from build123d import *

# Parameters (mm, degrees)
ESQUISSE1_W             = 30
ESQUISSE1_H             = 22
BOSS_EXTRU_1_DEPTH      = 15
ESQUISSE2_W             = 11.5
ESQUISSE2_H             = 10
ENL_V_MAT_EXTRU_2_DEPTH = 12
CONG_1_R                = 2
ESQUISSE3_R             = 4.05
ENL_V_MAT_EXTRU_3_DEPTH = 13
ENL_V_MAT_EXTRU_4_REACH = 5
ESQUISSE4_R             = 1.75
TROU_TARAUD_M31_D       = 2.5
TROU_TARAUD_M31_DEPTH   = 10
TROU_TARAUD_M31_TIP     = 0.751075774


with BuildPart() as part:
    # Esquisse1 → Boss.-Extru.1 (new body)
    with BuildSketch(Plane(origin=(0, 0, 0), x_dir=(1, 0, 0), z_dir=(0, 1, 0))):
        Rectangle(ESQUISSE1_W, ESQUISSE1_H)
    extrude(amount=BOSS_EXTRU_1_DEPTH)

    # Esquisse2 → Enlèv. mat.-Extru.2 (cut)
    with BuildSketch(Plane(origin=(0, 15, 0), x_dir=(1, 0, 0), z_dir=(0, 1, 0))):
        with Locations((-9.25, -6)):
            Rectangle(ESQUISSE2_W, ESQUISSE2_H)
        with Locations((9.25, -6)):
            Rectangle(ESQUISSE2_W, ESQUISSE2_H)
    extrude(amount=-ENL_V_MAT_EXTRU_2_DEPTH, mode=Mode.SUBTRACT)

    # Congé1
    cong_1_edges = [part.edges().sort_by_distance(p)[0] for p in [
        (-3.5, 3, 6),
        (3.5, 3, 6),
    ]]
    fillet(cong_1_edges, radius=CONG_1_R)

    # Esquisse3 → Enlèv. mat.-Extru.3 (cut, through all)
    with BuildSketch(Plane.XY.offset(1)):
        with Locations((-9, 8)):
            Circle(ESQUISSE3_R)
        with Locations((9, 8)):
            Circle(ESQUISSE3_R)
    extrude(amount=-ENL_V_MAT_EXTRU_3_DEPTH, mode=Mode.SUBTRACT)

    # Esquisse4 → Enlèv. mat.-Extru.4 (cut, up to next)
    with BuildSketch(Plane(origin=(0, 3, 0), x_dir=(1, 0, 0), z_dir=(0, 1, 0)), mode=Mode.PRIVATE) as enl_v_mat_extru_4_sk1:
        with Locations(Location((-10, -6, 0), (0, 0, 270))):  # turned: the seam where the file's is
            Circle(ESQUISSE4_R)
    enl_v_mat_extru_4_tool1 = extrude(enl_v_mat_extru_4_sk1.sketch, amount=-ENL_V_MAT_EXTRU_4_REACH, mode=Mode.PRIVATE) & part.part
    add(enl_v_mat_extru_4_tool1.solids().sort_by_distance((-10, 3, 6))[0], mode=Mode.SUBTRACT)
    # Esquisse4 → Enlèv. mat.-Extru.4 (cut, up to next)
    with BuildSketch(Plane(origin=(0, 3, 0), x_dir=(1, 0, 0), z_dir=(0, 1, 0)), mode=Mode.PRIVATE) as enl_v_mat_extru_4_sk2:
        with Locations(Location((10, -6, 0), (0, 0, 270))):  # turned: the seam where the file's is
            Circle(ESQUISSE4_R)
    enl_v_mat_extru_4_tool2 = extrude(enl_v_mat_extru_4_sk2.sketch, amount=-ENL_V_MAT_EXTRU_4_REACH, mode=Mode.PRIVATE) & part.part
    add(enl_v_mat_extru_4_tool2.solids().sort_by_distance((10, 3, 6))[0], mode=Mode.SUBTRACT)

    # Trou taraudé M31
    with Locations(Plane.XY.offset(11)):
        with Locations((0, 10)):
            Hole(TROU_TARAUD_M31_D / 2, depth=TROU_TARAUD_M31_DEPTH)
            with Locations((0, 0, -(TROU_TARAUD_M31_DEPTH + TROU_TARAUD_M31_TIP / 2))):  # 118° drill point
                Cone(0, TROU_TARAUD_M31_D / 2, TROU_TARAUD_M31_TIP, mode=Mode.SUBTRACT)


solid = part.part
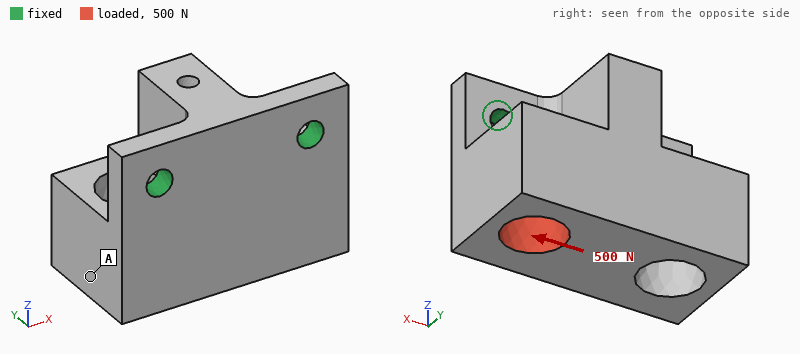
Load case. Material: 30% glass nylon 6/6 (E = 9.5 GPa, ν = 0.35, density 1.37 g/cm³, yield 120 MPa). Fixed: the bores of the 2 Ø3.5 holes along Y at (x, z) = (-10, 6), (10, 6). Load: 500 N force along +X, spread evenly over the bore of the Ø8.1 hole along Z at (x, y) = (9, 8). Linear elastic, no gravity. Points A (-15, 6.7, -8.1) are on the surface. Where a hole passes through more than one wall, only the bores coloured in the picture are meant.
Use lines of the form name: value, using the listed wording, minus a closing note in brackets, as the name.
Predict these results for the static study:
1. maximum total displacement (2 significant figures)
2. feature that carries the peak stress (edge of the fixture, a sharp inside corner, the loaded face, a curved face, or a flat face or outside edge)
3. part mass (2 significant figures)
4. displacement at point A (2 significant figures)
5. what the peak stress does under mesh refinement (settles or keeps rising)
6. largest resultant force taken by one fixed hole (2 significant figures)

maximum total displacement: 56 µm
feature that carries the peak stress: edge of the fixture
part mass: 8.0 g
displacement at point A: 38 µm
what the peak stress does under mesh refinement: keeps rising
largest resultant force taken by one fixed hole: 390 N
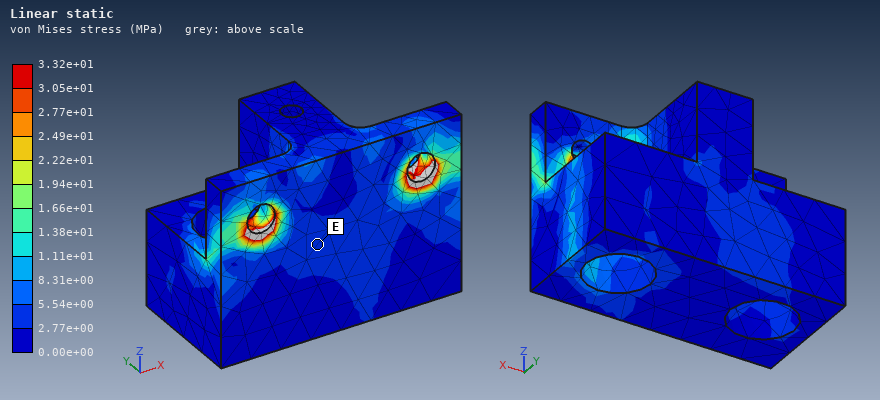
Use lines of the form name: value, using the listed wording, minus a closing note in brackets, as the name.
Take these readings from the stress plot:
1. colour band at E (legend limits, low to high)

colour band at E: 2.77e+00 to 5.54e+00 MPa
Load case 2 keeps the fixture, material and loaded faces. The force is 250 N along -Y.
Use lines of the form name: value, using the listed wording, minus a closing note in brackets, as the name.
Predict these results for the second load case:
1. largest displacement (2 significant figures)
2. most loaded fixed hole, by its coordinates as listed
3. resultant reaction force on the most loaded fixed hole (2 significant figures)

largest displacement: 0.25 mm
most loaded fixed hole, by its coordinates as listed: (10, 6)
resultant reaction force on the most loaded fixed hole: 240 N
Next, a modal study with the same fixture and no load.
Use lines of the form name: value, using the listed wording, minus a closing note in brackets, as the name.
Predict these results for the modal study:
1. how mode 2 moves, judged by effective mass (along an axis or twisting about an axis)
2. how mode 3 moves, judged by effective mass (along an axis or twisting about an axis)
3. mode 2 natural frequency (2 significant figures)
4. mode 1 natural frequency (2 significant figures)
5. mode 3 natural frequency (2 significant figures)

how mode 2 moves, judged by effective mass: along X
how mode 3 moves, judged by effective mass: along X
mode 2 natural frequency: 6400 Hz
mode 1 natural frequency: 2300 Hz
mode 3 natural frequency: 10 kHz
